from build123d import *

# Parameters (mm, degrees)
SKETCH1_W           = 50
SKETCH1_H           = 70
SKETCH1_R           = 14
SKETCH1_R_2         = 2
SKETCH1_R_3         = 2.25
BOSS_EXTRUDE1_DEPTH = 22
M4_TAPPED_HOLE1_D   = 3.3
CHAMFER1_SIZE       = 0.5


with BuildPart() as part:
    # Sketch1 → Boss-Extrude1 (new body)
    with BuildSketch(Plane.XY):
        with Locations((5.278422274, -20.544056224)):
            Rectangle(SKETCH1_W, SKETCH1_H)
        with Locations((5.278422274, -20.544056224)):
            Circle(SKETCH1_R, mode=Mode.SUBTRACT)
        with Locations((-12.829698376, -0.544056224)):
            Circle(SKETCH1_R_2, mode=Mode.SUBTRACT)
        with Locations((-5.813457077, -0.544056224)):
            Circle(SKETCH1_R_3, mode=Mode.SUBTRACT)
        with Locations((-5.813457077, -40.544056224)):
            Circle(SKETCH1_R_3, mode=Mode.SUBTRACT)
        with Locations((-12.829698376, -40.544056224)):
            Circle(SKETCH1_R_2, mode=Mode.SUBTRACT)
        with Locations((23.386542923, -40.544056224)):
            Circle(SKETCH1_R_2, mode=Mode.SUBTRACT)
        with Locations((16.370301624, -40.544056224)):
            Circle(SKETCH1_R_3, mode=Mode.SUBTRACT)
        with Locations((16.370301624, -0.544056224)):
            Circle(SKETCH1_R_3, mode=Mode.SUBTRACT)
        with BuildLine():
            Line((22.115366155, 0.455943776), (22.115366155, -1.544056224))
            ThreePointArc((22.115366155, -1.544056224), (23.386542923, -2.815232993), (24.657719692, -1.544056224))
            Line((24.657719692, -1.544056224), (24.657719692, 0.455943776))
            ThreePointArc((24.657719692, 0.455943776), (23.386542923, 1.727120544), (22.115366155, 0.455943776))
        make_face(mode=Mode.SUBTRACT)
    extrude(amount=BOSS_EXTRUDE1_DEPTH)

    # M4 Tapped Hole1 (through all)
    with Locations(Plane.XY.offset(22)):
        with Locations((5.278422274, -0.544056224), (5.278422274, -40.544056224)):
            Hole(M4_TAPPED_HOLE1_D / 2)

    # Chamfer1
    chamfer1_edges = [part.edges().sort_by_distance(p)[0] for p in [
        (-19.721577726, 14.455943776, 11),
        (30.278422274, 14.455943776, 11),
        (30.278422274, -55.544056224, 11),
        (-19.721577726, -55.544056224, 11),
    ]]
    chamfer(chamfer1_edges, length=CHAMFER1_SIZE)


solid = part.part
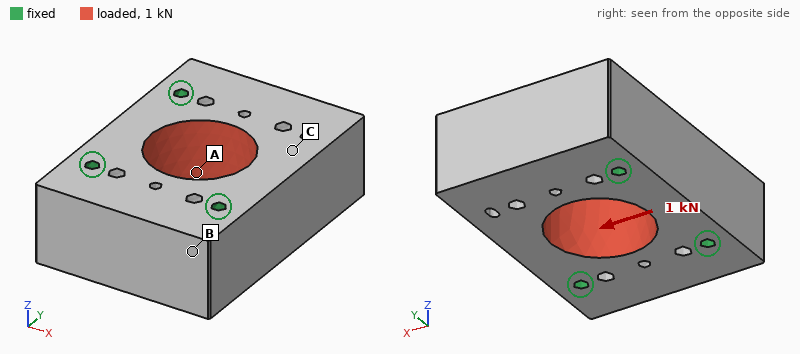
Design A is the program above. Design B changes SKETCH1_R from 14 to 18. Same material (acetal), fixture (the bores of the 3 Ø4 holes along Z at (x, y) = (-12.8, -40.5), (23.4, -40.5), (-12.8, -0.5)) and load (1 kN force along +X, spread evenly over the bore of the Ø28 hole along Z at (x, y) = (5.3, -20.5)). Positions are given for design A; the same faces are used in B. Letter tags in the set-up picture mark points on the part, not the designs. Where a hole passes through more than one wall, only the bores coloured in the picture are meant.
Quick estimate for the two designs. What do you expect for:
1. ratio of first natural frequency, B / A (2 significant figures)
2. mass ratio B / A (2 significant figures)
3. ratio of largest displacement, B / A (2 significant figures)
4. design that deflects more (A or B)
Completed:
0.94
0.85
1.7
B
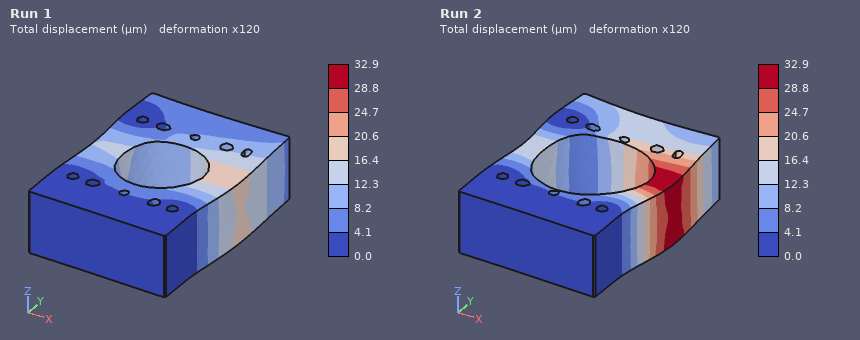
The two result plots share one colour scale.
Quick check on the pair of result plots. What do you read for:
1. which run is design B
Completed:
Run 2
